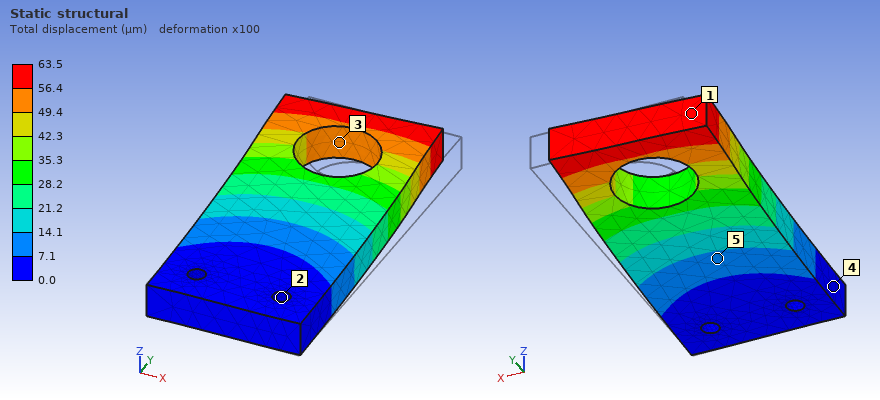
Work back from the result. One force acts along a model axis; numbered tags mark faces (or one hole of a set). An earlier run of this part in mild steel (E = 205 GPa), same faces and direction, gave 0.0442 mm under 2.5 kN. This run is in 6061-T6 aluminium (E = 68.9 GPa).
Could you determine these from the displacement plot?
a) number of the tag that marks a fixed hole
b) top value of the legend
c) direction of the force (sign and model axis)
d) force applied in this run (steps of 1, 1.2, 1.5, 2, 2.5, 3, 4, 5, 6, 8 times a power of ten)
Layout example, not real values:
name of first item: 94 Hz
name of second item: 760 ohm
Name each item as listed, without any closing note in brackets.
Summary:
number of the tag that marks a fixed hole: 2
top value of the legend: 63.5 µm
direction of the force: -X
force applied in this run: 1.2 kN
